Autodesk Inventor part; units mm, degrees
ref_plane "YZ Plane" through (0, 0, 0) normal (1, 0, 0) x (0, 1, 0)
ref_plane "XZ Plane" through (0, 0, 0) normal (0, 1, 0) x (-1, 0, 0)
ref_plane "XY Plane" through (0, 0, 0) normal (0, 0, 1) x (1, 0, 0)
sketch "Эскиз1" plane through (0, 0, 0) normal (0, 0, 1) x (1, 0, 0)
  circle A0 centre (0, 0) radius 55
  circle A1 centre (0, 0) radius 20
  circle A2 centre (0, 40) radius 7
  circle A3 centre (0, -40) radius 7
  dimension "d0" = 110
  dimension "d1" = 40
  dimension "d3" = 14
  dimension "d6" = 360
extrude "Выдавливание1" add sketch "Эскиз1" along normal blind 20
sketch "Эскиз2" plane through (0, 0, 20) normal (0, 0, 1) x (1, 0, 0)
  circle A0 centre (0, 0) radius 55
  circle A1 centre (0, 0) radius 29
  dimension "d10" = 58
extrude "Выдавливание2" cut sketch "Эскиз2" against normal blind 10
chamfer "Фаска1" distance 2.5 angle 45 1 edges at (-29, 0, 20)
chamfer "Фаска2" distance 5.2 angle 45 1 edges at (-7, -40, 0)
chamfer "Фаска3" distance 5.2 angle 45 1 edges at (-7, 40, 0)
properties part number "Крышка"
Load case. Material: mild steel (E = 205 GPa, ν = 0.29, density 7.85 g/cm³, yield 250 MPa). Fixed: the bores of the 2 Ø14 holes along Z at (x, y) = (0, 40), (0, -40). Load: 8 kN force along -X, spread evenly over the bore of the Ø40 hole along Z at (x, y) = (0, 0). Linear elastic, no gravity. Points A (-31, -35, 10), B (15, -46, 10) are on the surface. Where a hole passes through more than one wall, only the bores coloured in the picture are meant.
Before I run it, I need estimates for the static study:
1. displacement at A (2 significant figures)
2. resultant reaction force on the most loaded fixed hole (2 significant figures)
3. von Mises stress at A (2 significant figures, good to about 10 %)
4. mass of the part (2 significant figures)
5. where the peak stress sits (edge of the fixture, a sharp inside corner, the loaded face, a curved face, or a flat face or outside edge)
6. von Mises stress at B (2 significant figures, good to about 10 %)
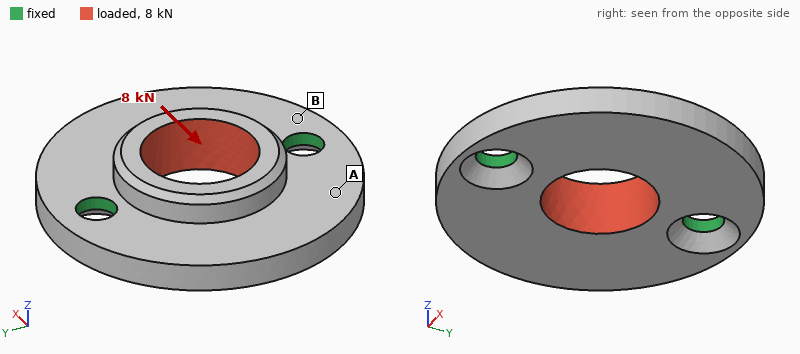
4.9 µm
4.0 kN
6.0 MPa
720 g
edge of the fixture
11 MPa
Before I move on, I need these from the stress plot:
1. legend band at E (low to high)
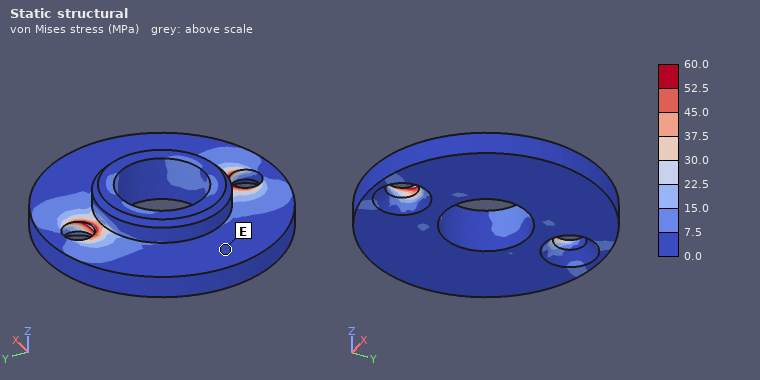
0.0 to 7.5 MPa
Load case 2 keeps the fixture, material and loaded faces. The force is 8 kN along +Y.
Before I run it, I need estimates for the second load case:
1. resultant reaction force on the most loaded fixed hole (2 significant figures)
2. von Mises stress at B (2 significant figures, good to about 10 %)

4.0 kN
5.9 MPa
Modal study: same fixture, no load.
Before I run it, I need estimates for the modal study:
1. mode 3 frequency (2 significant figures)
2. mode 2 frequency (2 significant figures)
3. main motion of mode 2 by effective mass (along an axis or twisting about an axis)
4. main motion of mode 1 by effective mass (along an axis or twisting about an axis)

6600 Hz
3400 Hz
along Z
twisting about Y
